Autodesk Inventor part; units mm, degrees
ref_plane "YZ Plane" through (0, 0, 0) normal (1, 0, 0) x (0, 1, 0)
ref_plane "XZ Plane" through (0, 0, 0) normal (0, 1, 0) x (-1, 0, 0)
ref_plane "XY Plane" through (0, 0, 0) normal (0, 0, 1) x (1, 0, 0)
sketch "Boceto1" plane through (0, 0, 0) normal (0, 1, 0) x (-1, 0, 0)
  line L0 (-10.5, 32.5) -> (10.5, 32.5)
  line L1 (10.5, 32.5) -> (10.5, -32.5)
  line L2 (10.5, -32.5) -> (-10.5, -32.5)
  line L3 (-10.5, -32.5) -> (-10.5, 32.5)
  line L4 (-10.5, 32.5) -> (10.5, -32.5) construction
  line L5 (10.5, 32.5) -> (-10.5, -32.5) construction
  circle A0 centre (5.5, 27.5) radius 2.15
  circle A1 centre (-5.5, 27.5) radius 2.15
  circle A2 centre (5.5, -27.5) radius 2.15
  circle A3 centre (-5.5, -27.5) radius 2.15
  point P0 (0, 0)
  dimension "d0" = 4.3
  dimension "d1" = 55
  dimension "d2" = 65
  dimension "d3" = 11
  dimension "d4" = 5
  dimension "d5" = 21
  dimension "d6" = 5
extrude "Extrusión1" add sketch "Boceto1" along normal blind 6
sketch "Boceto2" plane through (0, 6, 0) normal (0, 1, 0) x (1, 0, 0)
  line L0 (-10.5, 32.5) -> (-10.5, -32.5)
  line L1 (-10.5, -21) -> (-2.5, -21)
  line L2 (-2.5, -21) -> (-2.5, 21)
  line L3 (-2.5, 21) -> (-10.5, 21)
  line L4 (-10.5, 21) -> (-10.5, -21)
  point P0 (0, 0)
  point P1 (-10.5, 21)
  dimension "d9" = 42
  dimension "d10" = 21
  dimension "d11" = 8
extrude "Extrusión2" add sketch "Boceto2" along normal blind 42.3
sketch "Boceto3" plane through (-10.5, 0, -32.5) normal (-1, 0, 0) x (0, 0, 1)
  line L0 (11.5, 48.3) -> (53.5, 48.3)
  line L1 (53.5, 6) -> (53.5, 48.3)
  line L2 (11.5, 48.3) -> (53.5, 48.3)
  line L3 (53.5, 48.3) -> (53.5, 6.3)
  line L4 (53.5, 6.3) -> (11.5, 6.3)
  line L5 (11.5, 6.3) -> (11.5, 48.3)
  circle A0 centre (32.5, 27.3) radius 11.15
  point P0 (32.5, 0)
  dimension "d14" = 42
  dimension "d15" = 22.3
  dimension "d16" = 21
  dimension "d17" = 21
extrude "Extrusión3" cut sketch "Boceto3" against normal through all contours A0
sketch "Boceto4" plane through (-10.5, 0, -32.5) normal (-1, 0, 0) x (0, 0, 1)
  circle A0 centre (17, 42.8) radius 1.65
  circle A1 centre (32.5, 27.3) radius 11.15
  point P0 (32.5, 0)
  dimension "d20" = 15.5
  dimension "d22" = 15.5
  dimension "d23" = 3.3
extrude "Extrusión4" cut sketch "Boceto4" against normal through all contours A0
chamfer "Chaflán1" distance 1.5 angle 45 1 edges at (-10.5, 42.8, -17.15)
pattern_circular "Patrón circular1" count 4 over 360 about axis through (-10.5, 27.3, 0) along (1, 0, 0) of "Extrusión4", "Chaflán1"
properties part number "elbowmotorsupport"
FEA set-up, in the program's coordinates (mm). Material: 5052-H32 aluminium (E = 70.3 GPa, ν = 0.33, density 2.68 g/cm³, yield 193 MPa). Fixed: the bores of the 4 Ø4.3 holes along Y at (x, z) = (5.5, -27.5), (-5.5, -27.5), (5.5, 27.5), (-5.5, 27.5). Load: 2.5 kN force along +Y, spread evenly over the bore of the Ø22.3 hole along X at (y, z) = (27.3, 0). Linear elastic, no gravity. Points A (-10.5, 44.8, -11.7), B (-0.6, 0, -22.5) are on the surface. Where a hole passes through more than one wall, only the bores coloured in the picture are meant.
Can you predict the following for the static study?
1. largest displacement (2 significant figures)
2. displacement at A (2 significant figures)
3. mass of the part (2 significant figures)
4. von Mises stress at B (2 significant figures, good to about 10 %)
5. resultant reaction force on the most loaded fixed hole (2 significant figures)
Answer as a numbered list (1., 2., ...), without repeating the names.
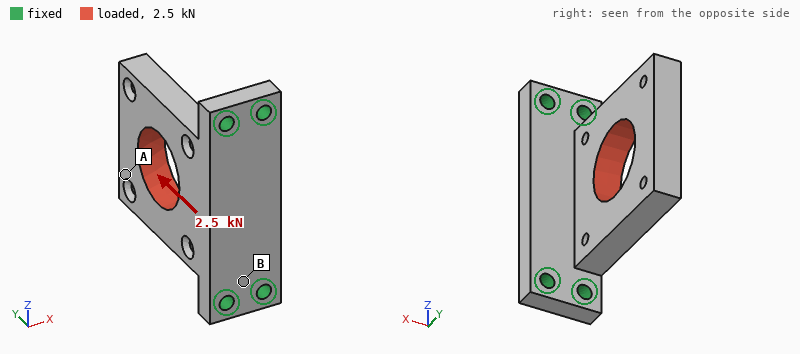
1. 47 µm
2. 44 µm
3. 50 g
4. 22 MPa
5. 1.3 kN
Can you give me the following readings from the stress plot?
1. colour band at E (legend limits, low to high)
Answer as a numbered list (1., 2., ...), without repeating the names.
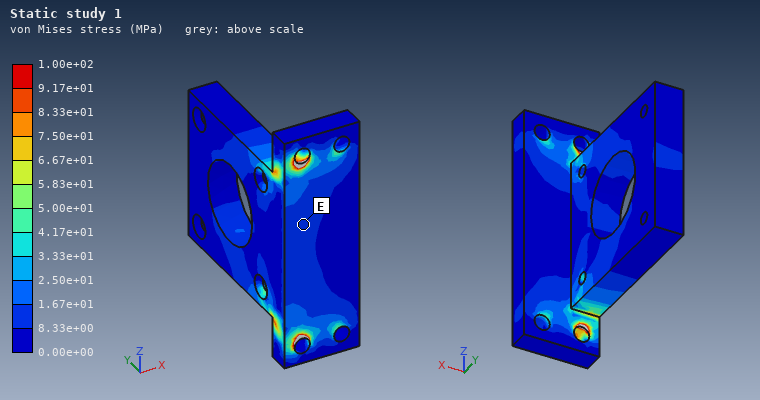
1. 8.33e+00 to 1.67e+01 MPa
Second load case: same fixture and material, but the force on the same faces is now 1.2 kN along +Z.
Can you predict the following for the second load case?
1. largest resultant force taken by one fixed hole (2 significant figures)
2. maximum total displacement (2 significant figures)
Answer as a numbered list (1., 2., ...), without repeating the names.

1. 680 N
2. 28 µm
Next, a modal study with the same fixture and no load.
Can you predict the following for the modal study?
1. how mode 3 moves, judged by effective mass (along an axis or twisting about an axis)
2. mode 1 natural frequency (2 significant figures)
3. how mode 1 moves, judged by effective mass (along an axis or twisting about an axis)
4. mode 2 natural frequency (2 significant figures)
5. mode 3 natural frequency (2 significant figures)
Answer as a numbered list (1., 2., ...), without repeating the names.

1. along Z
2. 2200 Hz
3. along X
4. 5900 Hz
5. 7100 Hz
